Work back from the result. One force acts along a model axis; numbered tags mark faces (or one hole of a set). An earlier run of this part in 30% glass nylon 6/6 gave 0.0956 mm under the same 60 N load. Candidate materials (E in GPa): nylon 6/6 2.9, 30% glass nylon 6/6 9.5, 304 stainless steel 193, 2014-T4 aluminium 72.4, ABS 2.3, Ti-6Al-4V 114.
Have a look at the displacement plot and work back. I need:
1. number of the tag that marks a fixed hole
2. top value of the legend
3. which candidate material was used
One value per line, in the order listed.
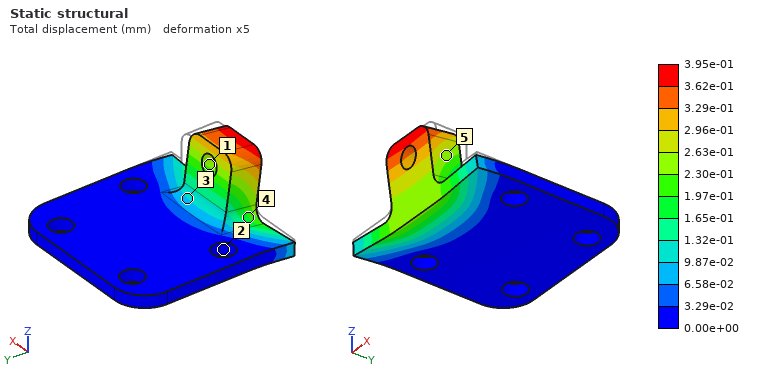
2
3.95e-01 mm
ABS
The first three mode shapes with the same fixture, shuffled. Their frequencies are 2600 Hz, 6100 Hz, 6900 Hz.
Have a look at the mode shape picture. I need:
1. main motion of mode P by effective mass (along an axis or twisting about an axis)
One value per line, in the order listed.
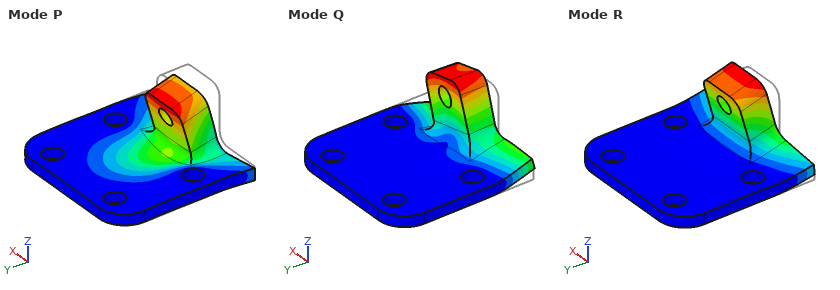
along Z
